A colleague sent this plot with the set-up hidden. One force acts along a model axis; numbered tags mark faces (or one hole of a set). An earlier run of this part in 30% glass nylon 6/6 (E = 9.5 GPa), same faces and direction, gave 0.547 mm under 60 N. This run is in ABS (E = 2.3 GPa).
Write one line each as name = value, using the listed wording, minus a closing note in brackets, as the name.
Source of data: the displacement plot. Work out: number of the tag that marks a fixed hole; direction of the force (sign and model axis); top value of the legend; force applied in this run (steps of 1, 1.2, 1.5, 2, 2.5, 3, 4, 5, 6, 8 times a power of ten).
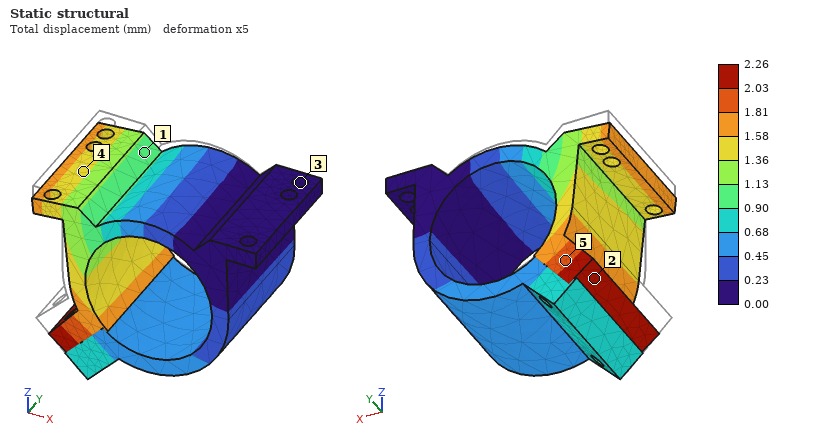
number of the tag that marks a fixed hole = 3
direction of the force = -Z
top value of the legend = 2.26 mm
force applied in this run = 60 N
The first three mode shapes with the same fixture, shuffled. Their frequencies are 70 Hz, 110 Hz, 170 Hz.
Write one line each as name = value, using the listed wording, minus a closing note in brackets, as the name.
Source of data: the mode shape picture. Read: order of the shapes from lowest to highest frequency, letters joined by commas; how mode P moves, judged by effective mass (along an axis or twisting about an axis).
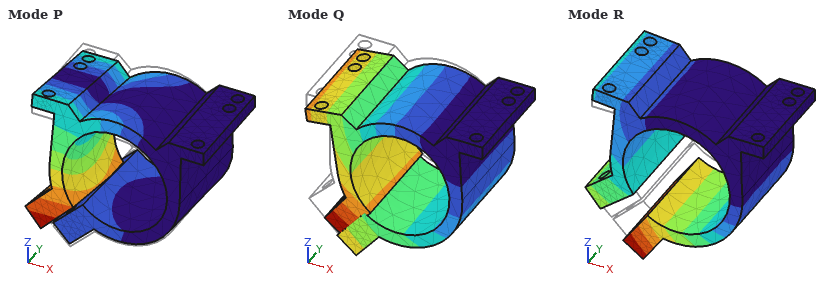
order of the shapes from lowest to highest frequency, letters joined by commas = Q, R, P
how mode P moves, judged by effective mass = along Y
